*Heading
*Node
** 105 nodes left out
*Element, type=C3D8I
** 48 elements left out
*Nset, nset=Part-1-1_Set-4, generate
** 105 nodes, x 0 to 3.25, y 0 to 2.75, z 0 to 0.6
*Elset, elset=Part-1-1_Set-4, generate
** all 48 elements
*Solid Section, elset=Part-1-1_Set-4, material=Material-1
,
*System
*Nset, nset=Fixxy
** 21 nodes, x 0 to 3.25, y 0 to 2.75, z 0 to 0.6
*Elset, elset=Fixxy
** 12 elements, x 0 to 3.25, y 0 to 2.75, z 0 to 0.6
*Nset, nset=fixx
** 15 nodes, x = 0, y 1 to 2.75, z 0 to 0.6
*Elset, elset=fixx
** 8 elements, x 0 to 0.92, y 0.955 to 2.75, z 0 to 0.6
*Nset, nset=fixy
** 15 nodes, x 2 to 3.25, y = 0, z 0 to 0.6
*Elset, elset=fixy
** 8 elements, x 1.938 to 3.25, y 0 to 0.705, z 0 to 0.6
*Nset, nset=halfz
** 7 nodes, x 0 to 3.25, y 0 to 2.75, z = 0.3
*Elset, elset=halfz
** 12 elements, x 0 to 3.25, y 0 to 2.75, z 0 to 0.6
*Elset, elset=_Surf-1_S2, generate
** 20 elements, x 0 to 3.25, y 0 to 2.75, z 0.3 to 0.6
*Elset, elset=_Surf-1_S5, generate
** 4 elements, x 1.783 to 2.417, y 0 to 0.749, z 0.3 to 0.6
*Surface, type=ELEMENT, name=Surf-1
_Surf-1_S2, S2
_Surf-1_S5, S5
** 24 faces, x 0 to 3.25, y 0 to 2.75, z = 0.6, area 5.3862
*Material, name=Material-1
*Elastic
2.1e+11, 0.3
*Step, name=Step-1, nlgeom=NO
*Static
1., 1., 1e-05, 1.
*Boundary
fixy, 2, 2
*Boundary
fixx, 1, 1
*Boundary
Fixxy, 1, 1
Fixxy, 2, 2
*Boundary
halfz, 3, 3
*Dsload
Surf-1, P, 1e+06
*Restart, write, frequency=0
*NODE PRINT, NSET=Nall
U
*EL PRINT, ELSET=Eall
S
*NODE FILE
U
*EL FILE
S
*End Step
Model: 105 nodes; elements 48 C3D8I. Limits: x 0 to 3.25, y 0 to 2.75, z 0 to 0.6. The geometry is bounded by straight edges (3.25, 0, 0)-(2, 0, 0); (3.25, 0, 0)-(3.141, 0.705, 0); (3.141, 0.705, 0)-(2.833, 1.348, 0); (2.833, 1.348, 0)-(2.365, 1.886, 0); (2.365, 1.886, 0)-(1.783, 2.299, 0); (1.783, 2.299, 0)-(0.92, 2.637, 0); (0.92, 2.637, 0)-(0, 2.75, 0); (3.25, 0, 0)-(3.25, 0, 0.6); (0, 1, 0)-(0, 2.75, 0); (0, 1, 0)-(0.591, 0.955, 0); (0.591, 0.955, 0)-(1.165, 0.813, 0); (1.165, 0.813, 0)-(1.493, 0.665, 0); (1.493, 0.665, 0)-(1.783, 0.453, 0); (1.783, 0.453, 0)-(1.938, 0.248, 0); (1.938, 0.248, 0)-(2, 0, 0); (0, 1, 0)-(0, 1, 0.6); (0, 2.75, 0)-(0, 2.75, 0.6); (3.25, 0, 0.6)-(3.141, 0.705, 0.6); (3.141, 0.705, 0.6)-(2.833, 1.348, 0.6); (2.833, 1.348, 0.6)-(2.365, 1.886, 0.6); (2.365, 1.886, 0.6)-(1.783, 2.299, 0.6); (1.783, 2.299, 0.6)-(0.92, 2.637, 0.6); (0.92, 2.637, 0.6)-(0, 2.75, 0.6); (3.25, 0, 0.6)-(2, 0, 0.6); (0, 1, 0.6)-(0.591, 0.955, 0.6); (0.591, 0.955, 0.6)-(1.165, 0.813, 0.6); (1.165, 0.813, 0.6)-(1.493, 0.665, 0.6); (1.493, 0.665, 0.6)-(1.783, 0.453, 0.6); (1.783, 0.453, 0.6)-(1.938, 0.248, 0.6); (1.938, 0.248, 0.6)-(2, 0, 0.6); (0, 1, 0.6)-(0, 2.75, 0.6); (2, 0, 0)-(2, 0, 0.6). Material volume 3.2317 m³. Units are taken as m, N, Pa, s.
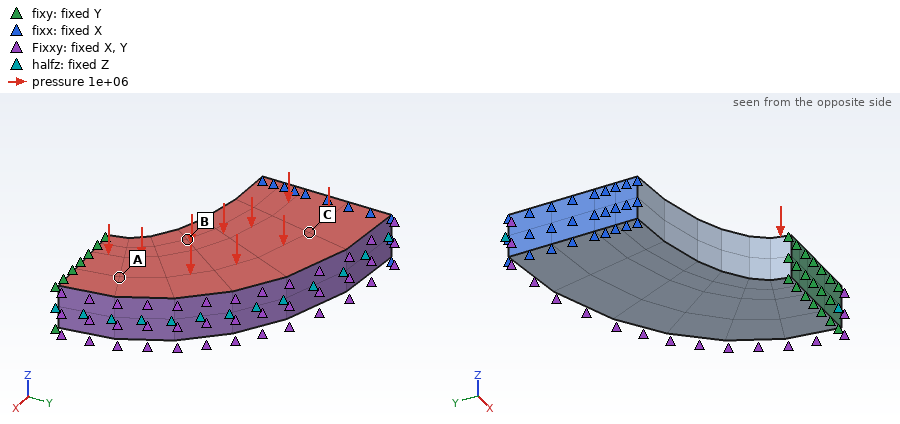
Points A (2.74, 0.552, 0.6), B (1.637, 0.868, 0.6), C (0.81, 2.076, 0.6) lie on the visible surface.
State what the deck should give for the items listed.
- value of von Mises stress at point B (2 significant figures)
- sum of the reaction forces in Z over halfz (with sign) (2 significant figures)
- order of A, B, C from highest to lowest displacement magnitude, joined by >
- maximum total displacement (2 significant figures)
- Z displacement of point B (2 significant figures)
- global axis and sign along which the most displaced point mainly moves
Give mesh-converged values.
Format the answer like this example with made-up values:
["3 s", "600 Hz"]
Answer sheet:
["4.3e+06 Pa", "5.4e+06 N", "B > C > A", "2.0e-04 m", "-1.1e-04 m", "-Z"]
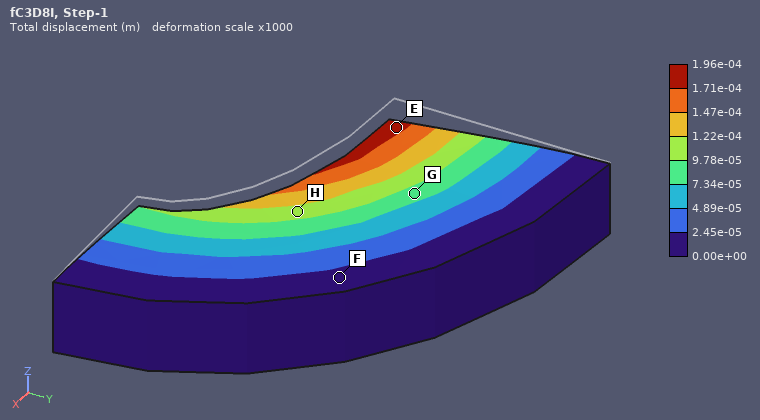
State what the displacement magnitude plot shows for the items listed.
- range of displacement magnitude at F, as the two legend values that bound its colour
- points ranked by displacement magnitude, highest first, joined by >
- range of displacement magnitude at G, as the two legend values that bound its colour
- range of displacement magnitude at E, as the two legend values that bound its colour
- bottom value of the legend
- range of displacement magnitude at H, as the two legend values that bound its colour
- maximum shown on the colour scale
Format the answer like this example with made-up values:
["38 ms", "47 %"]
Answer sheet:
["0.00e+00 to 2.45e-05 m", "E > H > G > F", "7.34e-05 to 9.78e-05 m", "1.71e-04 to 1.96e-04 m", "0.00e+00 m", "9.78e-05 to 1.22e-04 m", "1.96e-04 m"]
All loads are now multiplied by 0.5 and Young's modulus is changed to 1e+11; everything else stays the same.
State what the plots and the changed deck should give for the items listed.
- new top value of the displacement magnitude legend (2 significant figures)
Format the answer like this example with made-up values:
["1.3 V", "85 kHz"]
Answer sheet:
["2.1e-04 m"]
